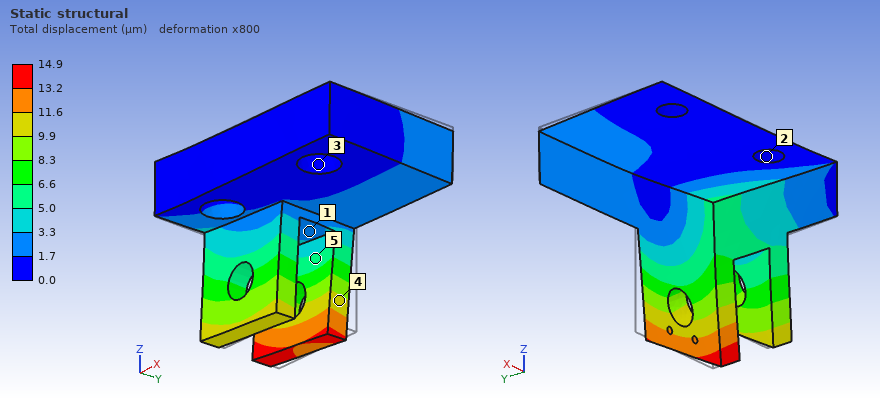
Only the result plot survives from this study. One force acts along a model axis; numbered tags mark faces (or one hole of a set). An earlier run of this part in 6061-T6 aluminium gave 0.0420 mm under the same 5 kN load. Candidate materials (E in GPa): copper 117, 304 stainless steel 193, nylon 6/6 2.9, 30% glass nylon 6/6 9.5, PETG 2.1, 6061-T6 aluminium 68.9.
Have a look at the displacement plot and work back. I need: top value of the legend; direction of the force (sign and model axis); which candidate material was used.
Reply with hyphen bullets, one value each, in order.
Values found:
- 14.9 µm
- -X
- 304 stainless steel
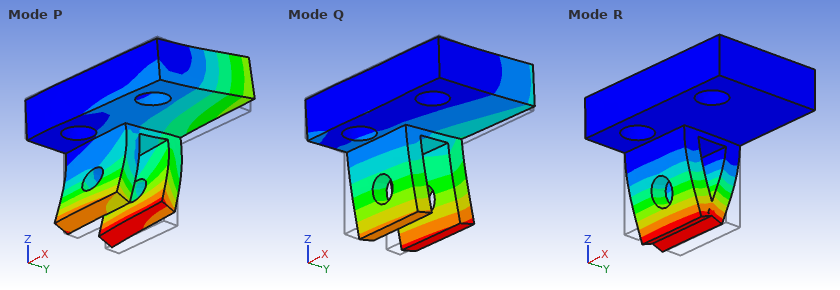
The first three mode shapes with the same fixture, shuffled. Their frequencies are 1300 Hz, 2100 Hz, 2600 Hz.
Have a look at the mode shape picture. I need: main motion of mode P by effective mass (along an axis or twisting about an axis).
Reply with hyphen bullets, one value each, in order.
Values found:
- along Z
